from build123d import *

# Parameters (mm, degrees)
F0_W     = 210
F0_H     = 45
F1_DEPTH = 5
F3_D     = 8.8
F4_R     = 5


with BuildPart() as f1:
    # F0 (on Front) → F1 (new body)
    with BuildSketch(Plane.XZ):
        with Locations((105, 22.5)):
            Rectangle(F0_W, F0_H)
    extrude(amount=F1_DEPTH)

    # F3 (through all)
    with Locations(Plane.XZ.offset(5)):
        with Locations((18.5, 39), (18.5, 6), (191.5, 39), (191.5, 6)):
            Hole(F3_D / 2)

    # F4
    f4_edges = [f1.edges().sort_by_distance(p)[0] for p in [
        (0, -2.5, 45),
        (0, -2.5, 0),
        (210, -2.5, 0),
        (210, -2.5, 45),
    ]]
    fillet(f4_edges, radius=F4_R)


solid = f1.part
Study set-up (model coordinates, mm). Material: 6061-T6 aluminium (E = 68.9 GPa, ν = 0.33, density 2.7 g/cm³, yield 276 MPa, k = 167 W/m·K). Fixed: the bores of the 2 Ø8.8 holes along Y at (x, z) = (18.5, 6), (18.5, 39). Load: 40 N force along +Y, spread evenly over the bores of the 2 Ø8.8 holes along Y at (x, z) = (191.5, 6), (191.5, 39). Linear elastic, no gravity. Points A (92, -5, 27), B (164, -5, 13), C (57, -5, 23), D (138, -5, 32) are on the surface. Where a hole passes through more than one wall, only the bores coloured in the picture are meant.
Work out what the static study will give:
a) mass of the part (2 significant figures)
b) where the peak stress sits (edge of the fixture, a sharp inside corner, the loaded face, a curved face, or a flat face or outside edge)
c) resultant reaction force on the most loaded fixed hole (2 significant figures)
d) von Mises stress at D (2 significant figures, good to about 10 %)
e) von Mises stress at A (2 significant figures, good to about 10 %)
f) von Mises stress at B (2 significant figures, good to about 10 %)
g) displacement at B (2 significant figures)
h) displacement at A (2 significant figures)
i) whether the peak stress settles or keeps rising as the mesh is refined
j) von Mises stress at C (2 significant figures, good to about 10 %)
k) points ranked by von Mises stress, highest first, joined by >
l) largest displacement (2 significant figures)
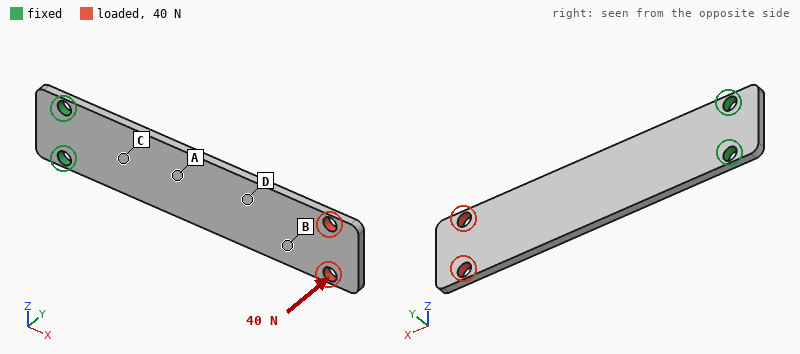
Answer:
120 g
edge of the fixture
20 N
12 MPa
21 MPa
6.0 MPa
1.5 mm
0.46 mm
keeps rising
28 MPa
C > A > D > B
2.4 mm
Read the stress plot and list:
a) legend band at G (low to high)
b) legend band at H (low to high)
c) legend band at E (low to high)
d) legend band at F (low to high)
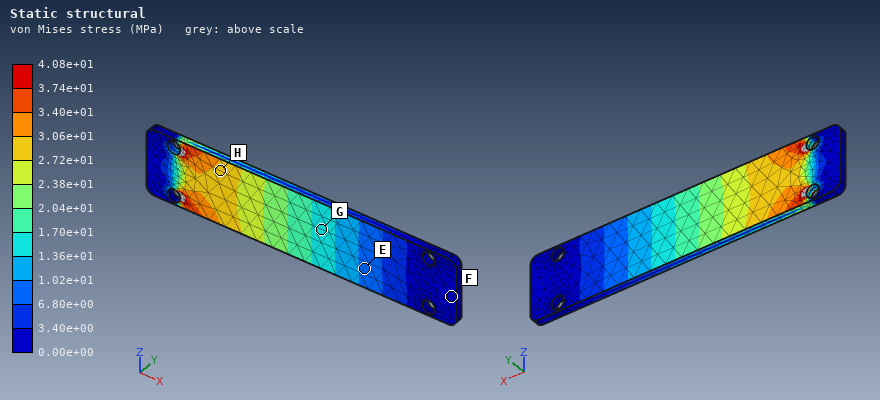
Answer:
1.36e+01 to 1.70e+01 MPa
2.72e+01 to 3.06e+01 MPa
6.80e+00 to 1.02e+01 MPa
0.00e+00 to 3.40e+00 MPa
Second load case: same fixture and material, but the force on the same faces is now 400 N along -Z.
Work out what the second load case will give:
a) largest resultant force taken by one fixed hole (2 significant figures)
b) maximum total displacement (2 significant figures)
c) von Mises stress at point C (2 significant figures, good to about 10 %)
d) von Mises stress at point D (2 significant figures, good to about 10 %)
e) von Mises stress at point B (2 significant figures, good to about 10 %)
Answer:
2.0 kN
0.31 mm
4.6 MPa
6.4 MPa
4.7 MPa
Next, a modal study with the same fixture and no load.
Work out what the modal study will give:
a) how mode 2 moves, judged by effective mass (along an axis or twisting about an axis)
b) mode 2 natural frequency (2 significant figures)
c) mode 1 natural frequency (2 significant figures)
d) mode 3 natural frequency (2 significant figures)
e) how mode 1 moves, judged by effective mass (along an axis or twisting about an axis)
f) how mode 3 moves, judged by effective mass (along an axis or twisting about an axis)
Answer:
along Y
720 Hz
120 Hz
960 Hz
along Y
twisting about X
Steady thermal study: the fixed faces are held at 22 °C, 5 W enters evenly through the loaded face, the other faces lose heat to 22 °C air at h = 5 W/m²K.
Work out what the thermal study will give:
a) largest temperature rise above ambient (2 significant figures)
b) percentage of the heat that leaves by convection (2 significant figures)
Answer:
21 K
20 %
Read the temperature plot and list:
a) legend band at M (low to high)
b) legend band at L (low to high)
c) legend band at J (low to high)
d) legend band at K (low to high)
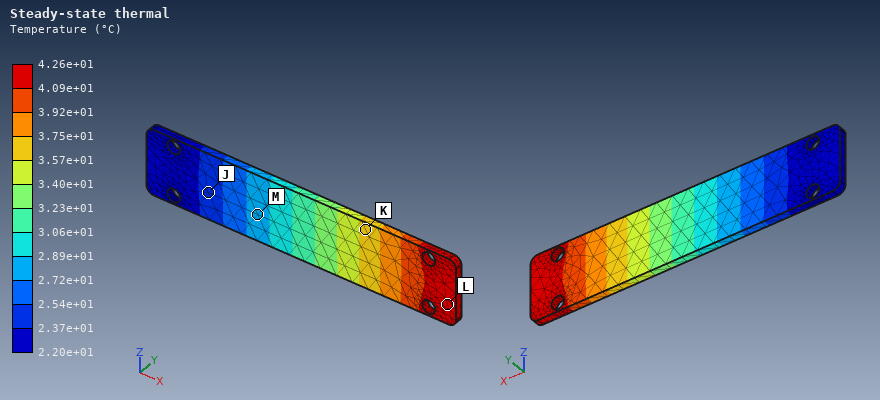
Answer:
2.72e+01 to 2.89e+01 °C
4.09e+01 to 4.26e+01 °C
2.37e+01 to 2.54e+01 °C
3.57e+01 to 3.75e+01 °C
